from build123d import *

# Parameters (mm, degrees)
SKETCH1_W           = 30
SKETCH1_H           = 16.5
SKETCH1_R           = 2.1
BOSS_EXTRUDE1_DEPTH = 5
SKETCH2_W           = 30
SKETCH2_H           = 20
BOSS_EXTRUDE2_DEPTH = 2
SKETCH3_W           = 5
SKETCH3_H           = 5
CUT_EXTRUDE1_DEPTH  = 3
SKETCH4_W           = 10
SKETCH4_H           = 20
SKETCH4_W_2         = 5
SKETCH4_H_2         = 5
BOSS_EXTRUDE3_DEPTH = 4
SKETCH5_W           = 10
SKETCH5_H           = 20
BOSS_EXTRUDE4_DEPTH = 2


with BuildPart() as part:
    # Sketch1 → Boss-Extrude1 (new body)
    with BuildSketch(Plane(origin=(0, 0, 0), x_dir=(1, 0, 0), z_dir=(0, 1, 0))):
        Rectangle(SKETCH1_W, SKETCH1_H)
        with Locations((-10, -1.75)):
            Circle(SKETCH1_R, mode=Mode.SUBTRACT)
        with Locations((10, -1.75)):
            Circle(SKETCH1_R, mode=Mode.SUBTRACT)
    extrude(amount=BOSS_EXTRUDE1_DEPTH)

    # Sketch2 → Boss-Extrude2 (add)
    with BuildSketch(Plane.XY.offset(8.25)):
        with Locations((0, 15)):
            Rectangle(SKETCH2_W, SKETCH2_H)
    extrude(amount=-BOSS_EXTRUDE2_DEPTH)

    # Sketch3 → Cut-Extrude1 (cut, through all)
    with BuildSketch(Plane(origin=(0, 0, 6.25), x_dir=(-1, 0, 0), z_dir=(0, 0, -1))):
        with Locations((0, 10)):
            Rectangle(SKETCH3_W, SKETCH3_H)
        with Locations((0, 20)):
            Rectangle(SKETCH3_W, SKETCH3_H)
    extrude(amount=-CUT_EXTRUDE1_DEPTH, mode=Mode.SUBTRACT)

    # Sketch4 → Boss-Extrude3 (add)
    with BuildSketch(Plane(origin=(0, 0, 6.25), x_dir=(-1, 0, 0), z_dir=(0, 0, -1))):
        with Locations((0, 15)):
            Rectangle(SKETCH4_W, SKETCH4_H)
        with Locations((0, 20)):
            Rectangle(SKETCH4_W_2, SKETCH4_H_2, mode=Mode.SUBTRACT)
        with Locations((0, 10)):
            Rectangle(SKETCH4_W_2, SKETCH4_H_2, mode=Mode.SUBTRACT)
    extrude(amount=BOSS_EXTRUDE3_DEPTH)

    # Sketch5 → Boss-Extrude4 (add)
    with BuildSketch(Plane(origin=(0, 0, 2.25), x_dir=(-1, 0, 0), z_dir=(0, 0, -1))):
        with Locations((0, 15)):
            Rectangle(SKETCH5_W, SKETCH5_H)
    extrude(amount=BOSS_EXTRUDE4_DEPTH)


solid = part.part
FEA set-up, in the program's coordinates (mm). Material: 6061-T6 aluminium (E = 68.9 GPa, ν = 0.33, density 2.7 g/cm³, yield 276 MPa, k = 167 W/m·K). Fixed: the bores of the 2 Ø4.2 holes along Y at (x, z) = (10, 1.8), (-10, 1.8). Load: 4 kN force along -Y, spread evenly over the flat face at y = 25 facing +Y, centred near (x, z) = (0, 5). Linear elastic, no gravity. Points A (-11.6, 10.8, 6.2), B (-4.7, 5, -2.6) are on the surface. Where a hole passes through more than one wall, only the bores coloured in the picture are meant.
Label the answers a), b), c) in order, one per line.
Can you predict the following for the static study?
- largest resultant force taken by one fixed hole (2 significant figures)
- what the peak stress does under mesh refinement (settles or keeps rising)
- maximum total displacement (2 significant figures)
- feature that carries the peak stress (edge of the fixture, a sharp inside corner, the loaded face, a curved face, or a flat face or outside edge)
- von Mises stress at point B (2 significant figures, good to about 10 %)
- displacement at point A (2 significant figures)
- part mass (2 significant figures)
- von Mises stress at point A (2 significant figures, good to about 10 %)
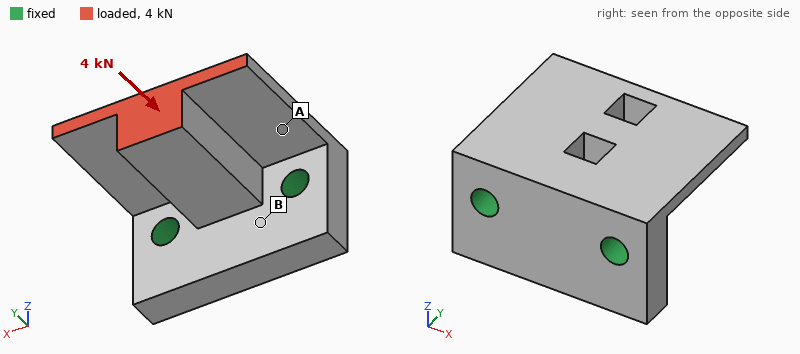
a) 2.0 kN
b) keeps rising
c) 43 µm
d) edge of the fixture
e) 21 MPa
f) 19 µm
g) 12 g
h) 55 MPa
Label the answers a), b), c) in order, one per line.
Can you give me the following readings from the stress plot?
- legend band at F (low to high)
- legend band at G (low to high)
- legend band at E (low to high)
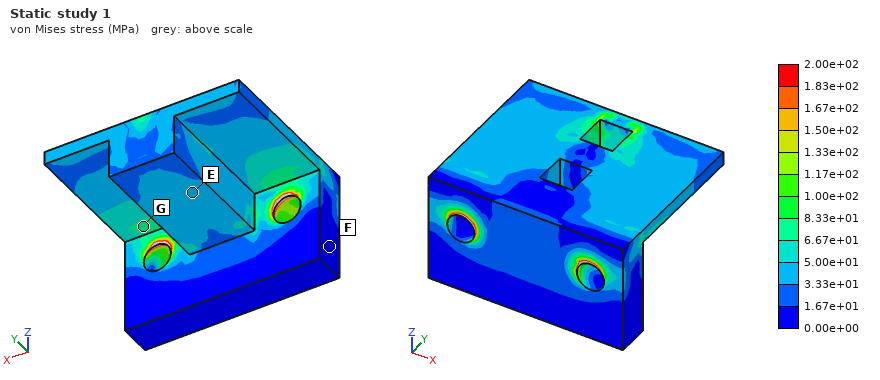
a) 0.00e+00 to 1.67e+01 MPa
b) 6.67e+01 to 8.33e+01 MPa
c) 3.33e+01 to 5.00e+01 MPa
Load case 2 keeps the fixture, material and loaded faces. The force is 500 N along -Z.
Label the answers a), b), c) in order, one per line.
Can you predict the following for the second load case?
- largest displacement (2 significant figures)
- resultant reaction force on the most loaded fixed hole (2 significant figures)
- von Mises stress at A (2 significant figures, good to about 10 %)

a) 0.13 mm
b) 250 N
c) 19 MPa
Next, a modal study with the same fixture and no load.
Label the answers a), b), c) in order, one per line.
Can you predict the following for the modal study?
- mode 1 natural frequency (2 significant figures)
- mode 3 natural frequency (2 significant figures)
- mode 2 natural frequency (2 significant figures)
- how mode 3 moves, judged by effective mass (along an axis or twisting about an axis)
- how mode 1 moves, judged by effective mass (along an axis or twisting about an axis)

a) 8300 Hz
b) 18 kHz
c) 12 kHz
d) along X
e) along Z
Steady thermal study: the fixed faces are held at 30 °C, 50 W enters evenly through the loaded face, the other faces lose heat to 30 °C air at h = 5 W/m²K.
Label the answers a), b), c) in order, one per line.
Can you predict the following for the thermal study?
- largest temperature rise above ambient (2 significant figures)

a) 79 K
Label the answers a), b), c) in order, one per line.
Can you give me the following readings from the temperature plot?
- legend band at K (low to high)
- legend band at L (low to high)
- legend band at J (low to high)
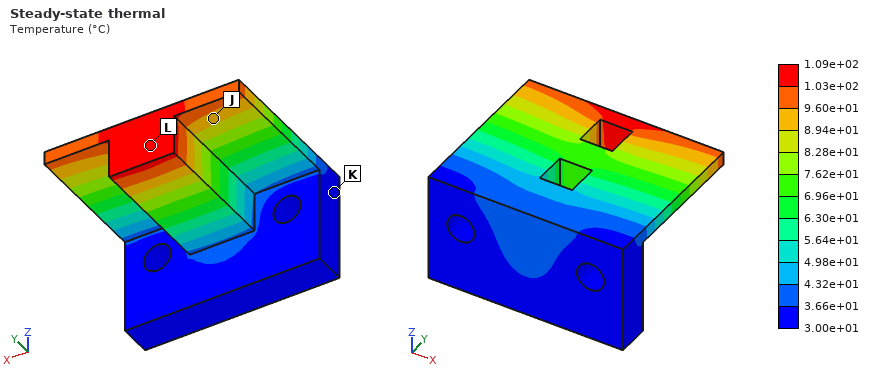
a) 3.00e+01 to 3.66e+01 °C
b) 1.03e+02 to 1.09e+02 °C
c) 8.94e+01 to 9.60e+01 °C
